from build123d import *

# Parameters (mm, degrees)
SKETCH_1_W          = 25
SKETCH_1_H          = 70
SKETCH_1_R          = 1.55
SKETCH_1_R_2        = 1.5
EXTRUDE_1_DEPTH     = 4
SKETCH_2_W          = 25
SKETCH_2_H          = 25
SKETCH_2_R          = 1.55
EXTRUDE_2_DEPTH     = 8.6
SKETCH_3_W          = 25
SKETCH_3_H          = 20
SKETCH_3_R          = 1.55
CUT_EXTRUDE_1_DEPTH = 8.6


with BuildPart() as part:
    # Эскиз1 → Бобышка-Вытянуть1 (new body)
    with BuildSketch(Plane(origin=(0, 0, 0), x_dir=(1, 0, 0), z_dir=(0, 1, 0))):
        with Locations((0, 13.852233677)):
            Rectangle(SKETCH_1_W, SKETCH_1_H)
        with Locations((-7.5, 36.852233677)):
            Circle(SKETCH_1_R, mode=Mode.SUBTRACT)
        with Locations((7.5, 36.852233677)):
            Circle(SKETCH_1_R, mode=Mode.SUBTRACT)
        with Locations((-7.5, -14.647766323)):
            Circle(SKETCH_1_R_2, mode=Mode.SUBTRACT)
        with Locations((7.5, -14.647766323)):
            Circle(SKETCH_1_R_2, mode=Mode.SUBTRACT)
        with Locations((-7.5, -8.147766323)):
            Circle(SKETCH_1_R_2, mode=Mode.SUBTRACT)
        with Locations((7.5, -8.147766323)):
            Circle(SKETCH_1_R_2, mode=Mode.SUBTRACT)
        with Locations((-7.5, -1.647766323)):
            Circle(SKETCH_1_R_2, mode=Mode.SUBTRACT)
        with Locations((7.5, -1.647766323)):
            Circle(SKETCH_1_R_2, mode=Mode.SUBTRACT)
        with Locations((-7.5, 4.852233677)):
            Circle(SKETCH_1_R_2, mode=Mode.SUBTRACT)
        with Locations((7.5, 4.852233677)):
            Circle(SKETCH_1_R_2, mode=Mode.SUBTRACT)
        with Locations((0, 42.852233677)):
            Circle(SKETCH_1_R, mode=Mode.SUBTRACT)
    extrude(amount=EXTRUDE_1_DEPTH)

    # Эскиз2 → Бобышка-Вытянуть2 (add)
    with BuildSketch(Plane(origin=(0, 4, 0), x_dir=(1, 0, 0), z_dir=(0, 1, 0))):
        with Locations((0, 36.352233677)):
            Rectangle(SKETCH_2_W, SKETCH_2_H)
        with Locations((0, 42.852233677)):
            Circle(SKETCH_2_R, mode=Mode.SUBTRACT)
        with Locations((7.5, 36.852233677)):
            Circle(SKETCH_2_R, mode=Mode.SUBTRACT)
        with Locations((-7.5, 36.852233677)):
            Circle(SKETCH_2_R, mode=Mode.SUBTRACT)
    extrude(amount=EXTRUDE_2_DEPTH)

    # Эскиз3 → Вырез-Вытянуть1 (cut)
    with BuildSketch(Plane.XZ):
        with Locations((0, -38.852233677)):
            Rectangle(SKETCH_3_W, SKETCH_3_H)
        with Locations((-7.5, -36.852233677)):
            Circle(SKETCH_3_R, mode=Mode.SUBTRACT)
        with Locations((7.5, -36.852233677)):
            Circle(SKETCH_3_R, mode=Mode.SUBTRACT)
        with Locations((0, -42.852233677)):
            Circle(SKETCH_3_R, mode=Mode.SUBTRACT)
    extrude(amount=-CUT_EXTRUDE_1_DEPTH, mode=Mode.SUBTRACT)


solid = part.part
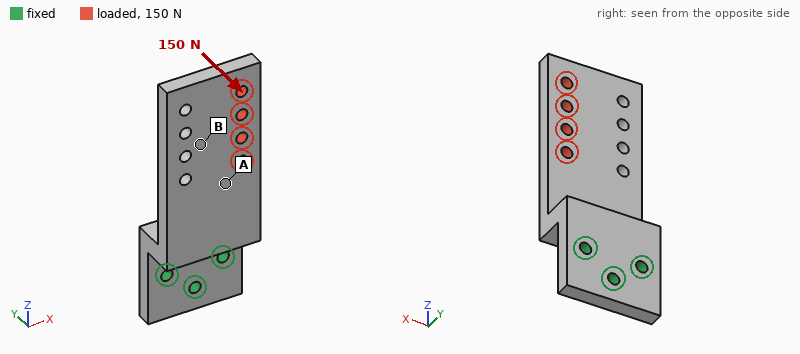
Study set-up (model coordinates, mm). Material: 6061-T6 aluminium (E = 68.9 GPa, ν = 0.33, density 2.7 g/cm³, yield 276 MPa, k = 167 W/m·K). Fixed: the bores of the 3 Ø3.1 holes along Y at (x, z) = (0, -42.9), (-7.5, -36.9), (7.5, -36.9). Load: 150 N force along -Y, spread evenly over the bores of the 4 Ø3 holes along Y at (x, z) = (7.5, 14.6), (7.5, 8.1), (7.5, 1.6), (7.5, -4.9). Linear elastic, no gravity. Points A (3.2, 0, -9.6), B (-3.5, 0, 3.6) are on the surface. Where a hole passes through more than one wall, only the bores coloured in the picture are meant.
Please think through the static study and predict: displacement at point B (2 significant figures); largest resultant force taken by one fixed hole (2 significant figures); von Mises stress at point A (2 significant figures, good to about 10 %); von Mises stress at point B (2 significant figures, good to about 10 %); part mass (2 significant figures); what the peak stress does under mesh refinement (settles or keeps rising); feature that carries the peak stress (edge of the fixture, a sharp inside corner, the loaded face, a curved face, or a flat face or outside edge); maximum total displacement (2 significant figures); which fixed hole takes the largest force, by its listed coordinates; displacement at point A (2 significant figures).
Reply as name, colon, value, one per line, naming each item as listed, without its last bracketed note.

displacement at point B: 0.38 mm
largest resultant force taken by one fixed hole: 220 N
von Mises stress at point A: 35 MPa
von Mises stress at point B: 15 MPa
part mass: 21 g
what the peak stress does under mesh refinement: keeps rising
feature that carries the peak stress: edge of the fixture
maximum total displacement: 0.69 mm
which fixed hole takes the largest force, by its listed coordinates: (7.5, -36.9)
displacement at point A: 0.22 mm
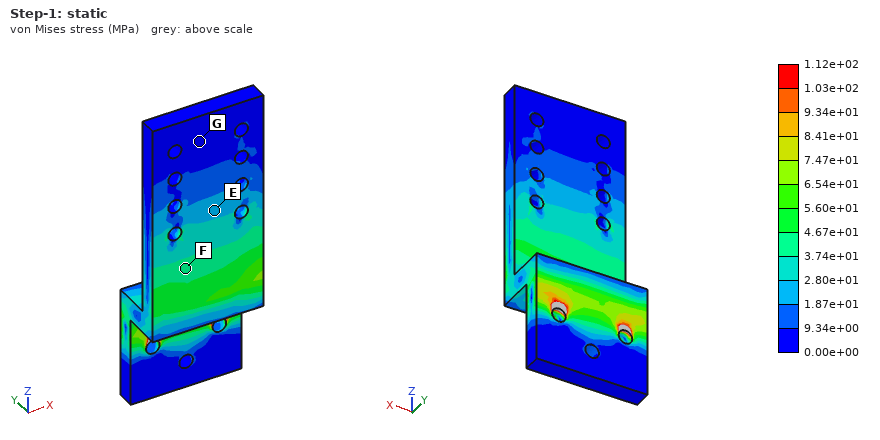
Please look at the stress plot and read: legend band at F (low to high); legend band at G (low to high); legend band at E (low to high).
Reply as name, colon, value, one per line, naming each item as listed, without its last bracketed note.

legend band at F: 3.74e+01 to 4.67e+01 MPa
legend band at G: 0.00e+00 to 9.34e+00 MPa
legend band at E: 1.87e+01 to 2.80e+01 MPa
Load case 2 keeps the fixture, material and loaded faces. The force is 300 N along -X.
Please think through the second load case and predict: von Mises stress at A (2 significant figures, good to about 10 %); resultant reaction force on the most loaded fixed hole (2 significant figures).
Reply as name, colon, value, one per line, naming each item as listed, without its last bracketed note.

von Mises stress at A: 5.4 MPa
resultant reaction force on the most loaded fixed hole: 760 N
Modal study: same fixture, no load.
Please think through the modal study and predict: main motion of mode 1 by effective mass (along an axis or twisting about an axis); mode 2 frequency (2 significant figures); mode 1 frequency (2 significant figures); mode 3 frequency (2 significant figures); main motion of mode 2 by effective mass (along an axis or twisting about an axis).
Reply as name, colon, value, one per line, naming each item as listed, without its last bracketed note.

main motion of mode 1 by effective mass: along Y
mode 2 frequency: 3200 Hz
mode 1 frequency: 980 Hz
mode 3 frequency: 4800 Hz
main motion of mode 2 by effective mass: along X
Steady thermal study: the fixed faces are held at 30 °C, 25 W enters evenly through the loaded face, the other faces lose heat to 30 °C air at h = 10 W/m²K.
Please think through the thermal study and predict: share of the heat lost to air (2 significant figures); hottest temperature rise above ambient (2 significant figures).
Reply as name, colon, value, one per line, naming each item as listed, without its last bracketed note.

share of the heat lost to air: 6.4 %
hottest temperature rise above ambient: 73 K
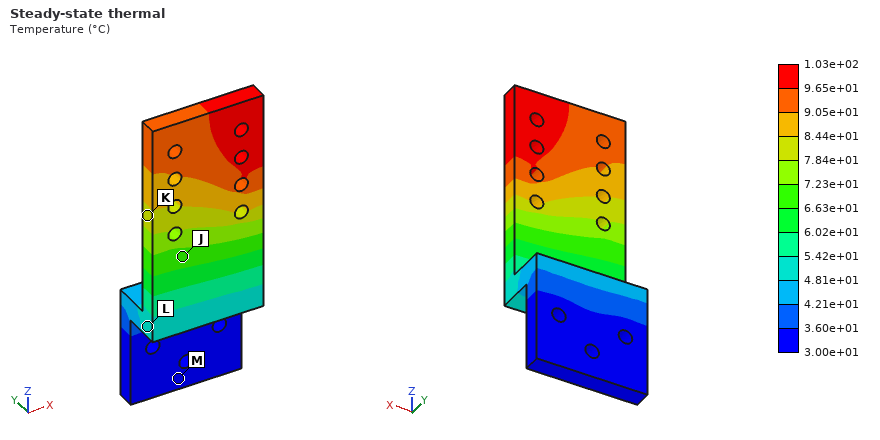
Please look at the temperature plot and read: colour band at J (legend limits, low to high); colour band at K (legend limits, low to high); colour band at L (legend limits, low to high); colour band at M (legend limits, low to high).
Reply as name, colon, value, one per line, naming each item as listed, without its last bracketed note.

colour band at J: 6.63e+01 to 7.23e+01 °C
colour band at K: 7.84e+01 to 8.44e+01 °C
colour band at L: 4.81e+01 to 5.42e+01 °C
colour band at M: 3.00e+01 to 3.60e+01 °C
